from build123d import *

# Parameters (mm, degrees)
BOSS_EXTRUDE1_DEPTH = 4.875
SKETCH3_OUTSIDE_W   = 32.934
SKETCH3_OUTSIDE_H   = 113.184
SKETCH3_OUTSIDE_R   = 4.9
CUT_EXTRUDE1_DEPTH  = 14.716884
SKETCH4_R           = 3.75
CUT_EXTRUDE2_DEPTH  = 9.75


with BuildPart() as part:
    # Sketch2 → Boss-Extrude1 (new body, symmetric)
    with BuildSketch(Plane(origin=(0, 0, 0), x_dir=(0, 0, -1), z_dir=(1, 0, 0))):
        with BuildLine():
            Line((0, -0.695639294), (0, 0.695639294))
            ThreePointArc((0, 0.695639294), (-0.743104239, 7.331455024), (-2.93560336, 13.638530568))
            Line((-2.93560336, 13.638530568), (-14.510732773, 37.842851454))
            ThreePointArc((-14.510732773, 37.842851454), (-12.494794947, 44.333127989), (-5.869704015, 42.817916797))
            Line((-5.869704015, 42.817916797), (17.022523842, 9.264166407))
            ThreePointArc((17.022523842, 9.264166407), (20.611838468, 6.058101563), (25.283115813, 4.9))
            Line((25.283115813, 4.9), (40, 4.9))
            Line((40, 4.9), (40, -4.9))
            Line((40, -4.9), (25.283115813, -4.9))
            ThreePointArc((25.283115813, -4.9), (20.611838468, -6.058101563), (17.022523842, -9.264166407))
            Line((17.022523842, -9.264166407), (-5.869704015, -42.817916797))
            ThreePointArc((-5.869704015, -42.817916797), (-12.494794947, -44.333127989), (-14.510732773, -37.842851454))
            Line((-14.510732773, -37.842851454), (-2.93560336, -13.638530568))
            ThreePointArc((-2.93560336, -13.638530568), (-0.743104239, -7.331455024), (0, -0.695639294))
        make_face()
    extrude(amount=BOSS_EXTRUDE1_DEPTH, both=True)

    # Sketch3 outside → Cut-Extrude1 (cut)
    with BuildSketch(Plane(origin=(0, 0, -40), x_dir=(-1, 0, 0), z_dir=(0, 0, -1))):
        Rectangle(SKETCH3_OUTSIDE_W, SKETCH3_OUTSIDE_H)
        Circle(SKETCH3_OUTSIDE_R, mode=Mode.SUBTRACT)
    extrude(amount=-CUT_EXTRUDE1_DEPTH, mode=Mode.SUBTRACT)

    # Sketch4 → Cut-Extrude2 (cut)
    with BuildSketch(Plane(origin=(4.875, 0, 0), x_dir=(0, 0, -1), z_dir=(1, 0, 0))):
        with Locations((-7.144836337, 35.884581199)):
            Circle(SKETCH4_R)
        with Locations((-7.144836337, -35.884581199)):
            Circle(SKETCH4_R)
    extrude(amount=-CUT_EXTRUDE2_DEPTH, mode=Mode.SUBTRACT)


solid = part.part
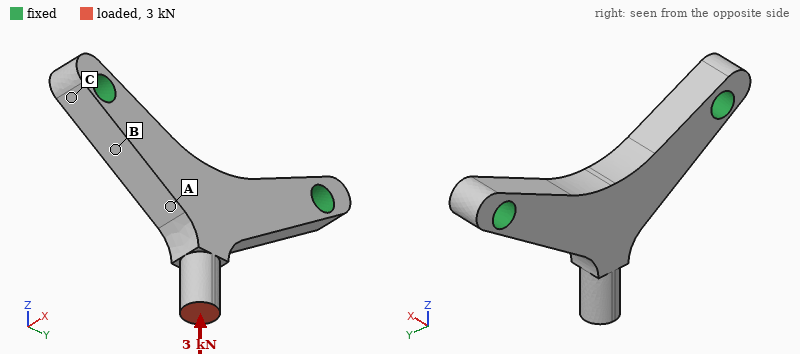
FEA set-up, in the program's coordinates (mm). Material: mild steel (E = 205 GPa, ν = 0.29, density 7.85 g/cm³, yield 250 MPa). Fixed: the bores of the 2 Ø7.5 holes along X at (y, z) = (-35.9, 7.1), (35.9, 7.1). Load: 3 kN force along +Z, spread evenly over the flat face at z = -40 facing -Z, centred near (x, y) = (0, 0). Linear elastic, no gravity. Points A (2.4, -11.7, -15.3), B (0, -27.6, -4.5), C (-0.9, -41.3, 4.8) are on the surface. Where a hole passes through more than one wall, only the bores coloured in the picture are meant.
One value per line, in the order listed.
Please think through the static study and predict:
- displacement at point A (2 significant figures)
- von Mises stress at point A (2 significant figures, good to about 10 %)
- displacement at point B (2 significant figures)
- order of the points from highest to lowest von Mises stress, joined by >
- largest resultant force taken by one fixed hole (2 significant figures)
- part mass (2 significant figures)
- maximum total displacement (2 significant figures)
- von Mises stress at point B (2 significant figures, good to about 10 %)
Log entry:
5.3 µm
31 MPa
1.6 µm
A > B > C
2.3 kN
110 g
10 µm
16 MPa
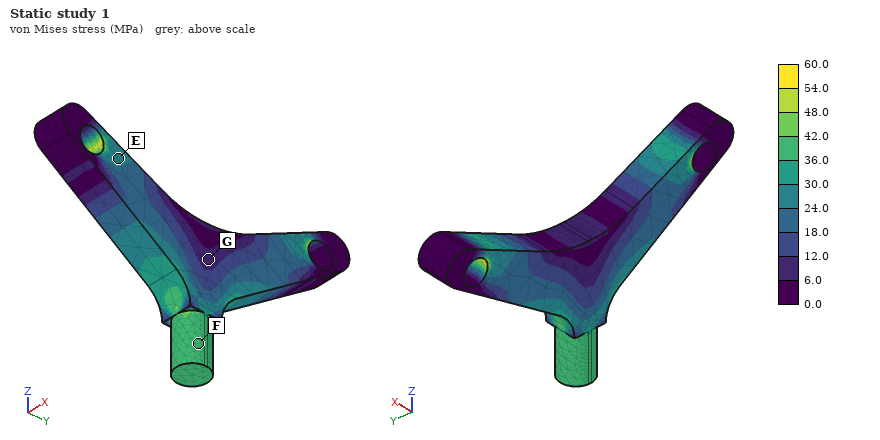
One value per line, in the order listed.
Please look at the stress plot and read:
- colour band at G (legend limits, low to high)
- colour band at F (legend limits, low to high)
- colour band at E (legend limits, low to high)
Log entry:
6.0 to 12.0 MPa
36.0 to 42.0 MPa
24.0 to 30.0 MPa
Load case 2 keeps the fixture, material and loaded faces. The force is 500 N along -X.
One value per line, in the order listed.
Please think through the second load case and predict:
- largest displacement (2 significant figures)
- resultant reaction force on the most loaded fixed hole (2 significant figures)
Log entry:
94 µm
250 N
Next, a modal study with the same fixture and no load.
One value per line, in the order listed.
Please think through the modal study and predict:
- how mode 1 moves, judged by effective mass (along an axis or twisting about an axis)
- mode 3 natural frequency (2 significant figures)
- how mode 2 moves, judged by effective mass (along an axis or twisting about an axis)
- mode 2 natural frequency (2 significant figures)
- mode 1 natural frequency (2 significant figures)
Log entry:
along X
13 kHz
along X
11 kHz
3800 Hz
